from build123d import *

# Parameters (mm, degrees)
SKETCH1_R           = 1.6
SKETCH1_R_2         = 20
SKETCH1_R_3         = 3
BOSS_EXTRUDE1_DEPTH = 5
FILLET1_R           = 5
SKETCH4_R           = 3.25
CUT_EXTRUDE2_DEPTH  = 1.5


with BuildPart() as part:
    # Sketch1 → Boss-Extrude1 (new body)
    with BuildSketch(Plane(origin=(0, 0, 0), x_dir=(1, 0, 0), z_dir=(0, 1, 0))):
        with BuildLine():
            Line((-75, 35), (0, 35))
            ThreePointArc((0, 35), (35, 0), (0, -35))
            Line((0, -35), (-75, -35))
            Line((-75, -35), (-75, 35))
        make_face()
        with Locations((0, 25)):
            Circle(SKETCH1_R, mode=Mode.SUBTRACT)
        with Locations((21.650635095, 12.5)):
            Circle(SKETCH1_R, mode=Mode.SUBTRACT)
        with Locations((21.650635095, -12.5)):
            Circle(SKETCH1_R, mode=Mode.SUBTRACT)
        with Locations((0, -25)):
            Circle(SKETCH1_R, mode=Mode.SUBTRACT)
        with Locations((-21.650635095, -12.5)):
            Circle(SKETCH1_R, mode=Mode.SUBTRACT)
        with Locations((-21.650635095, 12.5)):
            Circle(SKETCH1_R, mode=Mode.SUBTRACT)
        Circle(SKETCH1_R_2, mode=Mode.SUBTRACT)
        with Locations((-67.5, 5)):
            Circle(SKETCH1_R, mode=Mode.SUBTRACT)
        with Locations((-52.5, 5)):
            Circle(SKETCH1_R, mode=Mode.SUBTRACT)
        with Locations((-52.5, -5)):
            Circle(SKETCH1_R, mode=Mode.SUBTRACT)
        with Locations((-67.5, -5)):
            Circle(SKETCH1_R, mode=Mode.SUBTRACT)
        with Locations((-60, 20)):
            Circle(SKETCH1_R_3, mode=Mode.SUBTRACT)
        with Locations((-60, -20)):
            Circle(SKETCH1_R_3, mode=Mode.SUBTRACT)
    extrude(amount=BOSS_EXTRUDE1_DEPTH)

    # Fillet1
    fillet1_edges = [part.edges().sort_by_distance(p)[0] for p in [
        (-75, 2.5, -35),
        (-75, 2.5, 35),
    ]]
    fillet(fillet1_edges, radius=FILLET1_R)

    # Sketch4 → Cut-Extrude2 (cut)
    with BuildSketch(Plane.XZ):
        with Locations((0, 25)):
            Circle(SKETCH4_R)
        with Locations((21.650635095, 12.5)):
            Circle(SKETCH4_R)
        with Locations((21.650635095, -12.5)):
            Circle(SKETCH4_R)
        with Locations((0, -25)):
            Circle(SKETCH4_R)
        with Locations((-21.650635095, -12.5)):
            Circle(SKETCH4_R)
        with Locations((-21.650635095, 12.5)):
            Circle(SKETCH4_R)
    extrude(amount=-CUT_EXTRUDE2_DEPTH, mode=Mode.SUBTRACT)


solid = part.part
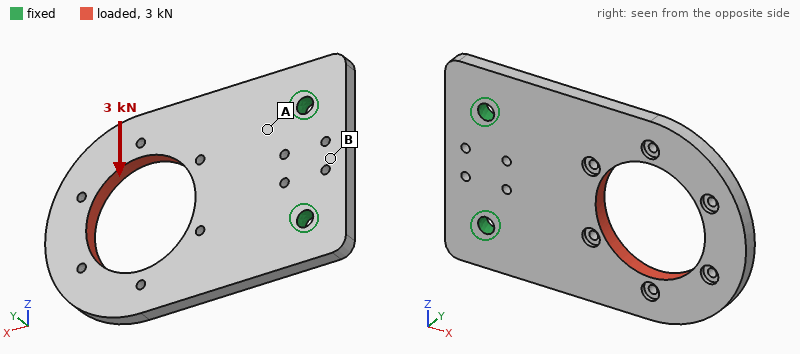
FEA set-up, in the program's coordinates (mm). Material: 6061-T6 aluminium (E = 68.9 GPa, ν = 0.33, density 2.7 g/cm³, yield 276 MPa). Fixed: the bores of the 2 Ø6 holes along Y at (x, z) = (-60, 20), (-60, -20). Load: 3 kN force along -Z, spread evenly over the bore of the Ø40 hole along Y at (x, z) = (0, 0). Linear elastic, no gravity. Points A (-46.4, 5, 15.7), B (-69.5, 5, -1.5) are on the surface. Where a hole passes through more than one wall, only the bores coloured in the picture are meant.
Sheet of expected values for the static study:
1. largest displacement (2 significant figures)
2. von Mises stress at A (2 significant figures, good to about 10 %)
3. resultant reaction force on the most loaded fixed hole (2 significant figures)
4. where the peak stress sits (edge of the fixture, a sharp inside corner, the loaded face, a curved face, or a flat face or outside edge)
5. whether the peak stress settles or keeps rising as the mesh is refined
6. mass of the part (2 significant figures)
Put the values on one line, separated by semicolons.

0.15 mm; 28 MPa; 4.4 kN; edge of the fixture; keeps rising; 77 g
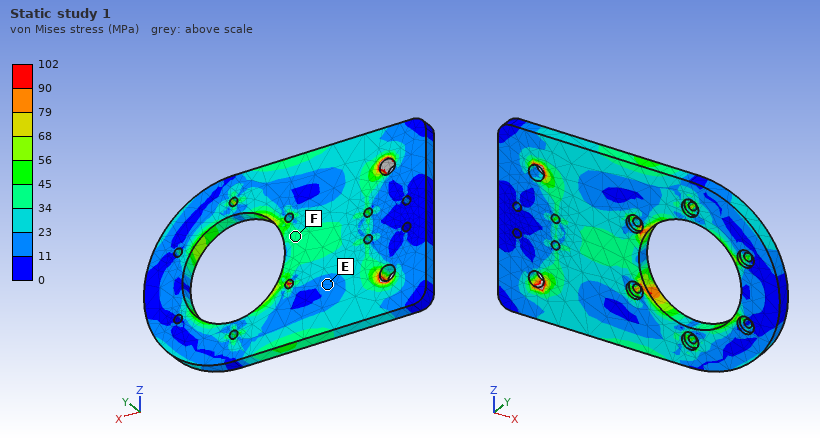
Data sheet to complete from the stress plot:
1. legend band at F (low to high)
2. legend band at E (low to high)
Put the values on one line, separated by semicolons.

34 to 45 MPa; 11 to 23 MPa
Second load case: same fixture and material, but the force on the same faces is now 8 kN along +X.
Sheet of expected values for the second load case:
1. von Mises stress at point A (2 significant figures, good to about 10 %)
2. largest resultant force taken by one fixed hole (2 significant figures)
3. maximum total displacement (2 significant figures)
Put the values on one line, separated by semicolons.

26 MPa; 4.0 kN; 73 µm
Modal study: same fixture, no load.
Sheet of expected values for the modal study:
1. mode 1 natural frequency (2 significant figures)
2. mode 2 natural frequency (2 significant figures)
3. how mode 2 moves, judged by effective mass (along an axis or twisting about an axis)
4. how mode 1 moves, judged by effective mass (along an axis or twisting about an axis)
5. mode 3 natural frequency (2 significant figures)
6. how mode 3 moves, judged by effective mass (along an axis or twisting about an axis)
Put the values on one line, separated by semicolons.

580 Hz; 1500 Hz; twisting about X; along Y; 2600 Hz; along Y
